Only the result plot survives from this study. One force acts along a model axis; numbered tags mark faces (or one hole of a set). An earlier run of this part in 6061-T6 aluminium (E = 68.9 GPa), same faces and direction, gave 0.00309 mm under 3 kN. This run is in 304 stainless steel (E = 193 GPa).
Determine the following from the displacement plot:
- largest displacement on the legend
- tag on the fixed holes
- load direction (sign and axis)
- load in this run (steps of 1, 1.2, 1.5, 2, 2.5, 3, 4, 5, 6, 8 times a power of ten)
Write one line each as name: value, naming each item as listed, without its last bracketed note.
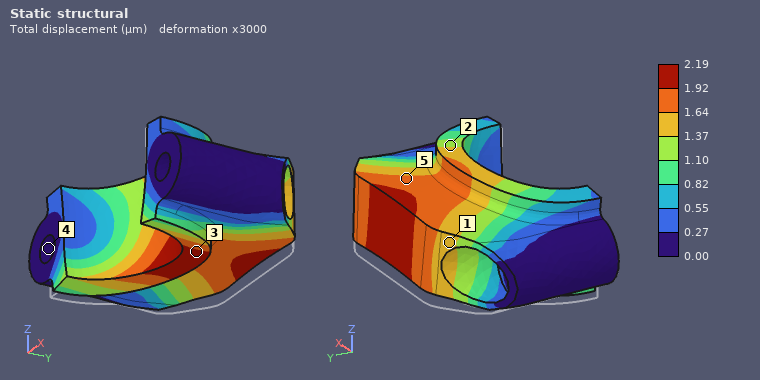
largest displacement on the legend: 2.19 µm
tag on the fixed holes: 4
load direction: +Z
load in this run: 6 kN
